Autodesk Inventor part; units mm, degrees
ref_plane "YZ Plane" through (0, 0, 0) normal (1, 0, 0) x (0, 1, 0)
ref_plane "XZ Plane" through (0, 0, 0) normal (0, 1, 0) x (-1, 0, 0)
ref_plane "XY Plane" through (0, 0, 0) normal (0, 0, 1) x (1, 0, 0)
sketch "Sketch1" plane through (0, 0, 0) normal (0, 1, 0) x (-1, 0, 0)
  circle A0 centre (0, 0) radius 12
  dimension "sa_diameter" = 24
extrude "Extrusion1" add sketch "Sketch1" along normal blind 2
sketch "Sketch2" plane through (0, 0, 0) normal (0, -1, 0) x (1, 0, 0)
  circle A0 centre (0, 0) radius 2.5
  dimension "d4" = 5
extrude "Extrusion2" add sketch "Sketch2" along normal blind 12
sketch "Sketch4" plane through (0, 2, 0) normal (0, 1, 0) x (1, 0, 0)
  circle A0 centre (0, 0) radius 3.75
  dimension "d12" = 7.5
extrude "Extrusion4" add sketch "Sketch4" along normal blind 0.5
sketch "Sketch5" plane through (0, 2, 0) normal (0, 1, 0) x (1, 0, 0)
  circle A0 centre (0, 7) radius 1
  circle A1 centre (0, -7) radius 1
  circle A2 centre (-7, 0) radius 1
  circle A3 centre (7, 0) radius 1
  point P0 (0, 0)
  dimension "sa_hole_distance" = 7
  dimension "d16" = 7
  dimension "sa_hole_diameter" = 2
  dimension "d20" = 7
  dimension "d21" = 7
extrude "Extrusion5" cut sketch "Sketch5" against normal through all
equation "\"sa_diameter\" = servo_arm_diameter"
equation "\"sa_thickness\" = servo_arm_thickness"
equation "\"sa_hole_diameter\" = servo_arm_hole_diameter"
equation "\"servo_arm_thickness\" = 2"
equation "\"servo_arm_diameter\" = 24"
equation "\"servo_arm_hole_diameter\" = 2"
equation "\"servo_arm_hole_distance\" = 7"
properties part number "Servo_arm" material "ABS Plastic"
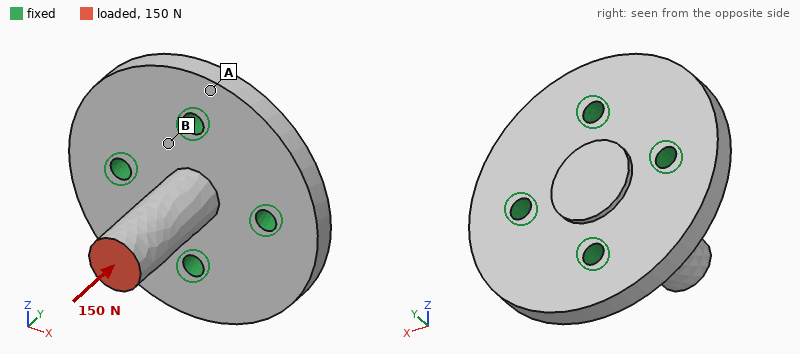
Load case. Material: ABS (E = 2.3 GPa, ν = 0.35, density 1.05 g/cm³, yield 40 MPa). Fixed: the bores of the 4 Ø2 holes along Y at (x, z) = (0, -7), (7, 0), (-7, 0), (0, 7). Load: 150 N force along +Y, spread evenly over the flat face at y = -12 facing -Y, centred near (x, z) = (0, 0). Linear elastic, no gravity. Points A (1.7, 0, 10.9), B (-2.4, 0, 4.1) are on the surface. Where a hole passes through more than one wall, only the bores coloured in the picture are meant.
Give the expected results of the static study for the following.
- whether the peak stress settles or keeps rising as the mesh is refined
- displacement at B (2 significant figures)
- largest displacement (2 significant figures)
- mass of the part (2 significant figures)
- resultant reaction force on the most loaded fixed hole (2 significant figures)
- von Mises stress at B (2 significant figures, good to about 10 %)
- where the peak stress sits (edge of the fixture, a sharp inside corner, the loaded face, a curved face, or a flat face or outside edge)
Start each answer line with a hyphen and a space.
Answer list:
- keeps rising
- 23 µm
- 87 µm
- 1.2 g
- 38 N
- 5.0 MPa
- edge of the fixture
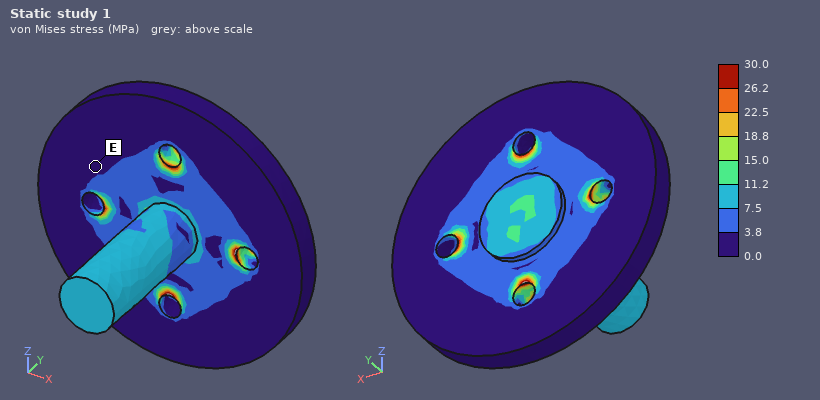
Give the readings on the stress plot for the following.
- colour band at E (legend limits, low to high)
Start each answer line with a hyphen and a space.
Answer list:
- 0.0 to 3.8 MPa
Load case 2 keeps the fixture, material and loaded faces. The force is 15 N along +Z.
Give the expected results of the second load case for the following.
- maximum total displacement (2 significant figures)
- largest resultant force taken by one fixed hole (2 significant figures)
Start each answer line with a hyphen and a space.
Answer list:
- 0.22 mm
- 17 N
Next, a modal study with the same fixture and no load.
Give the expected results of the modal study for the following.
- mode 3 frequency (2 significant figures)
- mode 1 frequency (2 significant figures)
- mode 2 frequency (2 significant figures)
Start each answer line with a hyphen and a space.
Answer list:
- 11 kHz
- 4900 Hz
- 5000 Hz
